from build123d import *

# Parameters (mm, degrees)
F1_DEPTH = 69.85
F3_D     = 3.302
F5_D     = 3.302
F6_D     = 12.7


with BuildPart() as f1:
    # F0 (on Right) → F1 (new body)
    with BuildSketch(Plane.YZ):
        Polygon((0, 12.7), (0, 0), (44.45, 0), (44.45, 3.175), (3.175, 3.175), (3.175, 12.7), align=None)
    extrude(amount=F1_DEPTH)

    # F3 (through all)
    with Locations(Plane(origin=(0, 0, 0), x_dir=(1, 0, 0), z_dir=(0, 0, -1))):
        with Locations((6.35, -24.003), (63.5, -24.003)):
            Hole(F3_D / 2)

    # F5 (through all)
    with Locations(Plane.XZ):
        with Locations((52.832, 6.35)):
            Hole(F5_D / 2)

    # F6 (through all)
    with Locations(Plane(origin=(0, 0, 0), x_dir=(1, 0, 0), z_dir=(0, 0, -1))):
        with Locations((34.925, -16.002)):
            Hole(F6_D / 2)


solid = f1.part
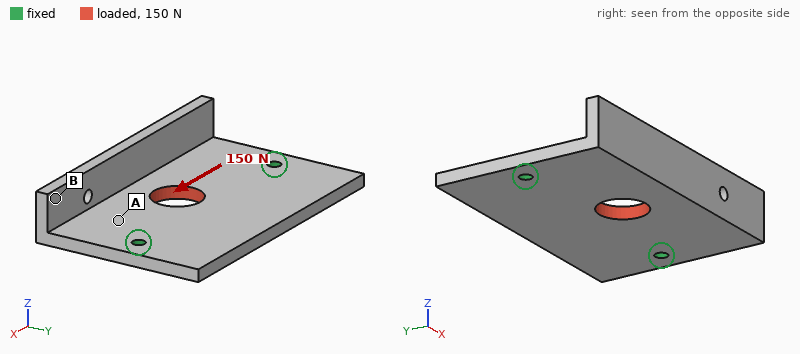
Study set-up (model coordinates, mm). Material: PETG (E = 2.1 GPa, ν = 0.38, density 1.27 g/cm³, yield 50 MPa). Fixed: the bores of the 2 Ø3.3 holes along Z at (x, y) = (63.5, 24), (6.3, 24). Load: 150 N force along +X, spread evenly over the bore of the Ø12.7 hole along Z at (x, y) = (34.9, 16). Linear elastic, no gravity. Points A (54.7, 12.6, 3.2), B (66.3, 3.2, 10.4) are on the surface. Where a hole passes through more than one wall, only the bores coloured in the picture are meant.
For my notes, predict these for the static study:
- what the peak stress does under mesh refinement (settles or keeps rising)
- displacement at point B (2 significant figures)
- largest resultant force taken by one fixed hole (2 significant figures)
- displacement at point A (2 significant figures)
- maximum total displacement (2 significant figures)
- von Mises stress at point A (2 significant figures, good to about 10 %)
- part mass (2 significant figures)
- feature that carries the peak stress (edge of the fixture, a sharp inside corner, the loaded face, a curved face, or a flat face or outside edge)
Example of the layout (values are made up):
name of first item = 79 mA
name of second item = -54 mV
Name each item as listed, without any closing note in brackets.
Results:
what the peak stress does under mesh refinement = keeps rising
displacement at point B = 19 µm
largest resultant force taken by one fixed hole = 78 N
displacement at point A = 15 µm
maximum total displacement = 26 µm
von Mises stress at point A = 0.91 MPa
part mass = 15 g
feature that carries the peak stress = edge of the fixture
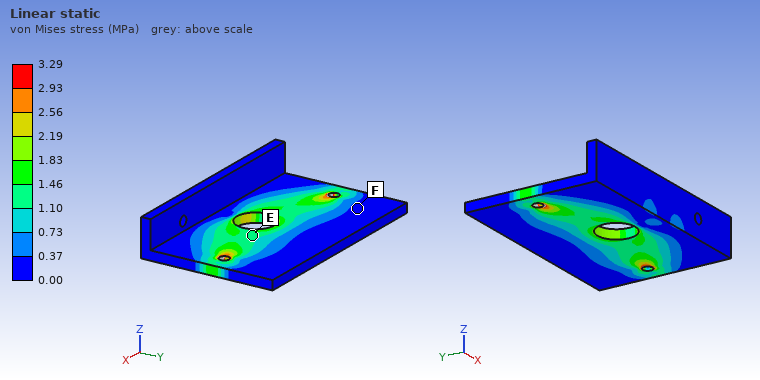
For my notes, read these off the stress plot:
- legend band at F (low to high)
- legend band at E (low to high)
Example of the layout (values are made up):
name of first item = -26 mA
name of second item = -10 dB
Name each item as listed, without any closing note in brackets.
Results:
legend band at F = 0.00 to 0.37 MPa
legend band at E = 1.10 to 1.46 MPa
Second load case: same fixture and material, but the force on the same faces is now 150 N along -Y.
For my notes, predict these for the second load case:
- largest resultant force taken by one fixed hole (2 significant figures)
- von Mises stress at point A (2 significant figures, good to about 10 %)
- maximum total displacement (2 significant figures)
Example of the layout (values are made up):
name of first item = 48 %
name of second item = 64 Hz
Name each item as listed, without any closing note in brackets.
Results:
largest resultant force taken by one fixed hole = 75 N
von Mises stress at point A = 1.3 MPa
maximum total displacement = 50 µm
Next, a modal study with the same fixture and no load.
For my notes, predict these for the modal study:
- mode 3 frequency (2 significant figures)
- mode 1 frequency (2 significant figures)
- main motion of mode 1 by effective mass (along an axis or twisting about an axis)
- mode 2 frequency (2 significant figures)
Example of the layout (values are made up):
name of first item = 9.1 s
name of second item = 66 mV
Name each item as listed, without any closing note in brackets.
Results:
mode 3 frequency = 990 Hz
mode 1 frequency = 540 Hz
main motion of mode 1 by effective mass = along Z
mode 2 frequency = 960 Hz
